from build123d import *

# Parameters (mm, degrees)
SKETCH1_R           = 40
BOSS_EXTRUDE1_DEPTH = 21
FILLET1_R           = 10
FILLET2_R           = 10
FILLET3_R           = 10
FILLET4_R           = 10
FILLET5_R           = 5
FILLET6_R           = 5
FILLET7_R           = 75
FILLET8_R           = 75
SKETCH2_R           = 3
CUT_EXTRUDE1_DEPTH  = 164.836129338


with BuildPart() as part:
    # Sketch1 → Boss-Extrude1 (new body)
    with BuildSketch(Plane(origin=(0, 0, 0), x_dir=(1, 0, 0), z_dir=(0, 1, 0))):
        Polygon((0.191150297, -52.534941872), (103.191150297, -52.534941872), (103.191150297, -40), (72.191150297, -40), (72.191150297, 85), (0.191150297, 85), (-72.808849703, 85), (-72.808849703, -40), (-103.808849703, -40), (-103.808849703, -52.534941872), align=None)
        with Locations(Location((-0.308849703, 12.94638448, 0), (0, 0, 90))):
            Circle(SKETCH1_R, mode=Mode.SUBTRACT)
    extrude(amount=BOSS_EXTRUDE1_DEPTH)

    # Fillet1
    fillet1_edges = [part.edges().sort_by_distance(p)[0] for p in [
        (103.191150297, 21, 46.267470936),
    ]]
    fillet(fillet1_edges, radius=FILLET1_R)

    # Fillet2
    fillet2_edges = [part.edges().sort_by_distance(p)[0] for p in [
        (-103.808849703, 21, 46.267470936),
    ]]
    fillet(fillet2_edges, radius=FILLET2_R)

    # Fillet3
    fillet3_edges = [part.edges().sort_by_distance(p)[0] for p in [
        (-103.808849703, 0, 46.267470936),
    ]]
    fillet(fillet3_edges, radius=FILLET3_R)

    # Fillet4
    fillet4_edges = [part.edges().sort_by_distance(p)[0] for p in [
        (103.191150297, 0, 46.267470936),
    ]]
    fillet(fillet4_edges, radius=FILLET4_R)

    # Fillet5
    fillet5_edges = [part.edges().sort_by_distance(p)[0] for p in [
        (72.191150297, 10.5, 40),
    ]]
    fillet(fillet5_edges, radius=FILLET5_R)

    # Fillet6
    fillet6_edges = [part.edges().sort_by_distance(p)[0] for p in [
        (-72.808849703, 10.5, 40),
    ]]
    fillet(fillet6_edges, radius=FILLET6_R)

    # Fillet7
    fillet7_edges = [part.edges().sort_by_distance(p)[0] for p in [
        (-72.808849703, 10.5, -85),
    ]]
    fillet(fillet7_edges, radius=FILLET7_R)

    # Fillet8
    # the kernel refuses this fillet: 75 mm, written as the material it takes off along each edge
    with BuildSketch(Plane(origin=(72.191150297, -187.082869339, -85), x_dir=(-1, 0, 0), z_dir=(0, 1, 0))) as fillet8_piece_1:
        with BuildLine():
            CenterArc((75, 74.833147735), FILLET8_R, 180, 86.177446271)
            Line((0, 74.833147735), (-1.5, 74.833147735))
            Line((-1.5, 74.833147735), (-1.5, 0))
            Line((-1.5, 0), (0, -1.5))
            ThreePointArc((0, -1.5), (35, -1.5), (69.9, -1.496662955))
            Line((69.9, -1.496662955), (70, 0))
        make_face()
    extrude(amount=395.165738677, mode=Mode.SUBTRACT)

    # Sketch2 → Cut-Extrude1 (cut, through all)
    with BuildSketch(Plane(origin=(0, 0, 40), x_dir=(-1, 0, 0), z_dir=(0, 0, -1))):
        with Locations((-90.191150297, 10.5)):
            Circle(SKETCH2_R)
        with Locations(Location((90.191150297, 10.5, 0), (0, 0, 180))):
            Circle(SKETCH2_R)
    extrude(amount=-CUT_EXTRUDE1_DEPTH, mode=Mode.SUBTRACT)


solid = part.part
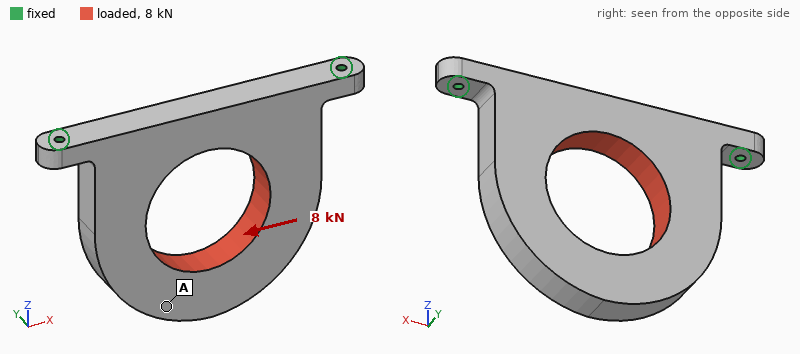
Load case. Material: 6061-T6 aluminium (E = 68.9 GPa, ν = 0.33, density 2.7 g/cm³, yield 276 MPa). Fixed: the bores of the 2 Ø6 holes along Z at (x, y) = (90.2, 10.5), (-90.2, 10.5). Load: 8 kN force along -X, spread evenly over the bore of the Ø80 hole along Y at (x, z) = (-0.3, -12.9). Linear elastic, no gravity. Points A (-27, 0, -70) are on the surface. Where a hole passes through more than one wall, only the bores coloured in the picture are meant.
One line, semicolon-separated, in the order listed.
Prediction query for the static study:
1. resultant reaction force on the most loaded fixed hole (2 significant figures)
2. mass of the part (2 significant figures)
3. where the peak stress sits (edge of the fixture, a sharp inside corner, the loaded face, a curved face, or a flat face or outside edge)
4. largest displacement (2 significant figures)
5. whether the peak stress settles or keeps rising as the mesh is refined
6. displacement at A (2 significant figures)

5.0 kN; 750 g; edge of the fixture; 68 µm; keeps rising; 67 µm
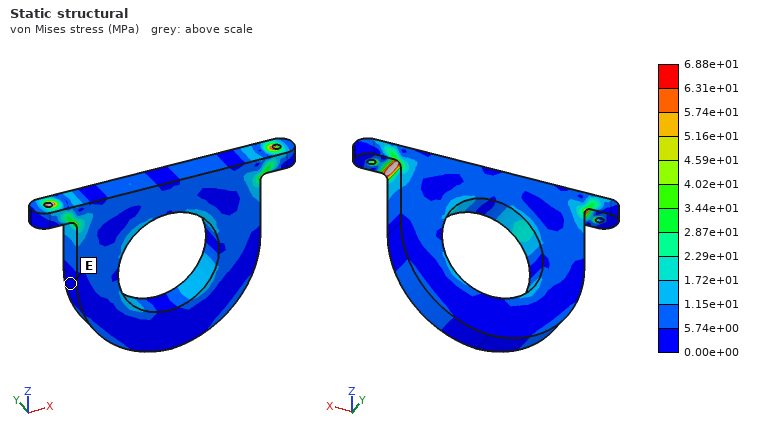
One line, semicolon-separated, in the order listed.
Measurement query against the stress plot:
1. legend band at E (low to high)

0.00e+00 to 5.74e+00 MPa
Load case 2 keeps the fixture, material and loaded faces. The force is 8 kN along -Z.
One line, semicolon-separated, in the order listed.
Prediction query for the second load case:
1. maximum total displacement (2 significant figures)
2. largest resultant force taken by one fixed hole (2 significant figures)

53 µm; 4.7 kN
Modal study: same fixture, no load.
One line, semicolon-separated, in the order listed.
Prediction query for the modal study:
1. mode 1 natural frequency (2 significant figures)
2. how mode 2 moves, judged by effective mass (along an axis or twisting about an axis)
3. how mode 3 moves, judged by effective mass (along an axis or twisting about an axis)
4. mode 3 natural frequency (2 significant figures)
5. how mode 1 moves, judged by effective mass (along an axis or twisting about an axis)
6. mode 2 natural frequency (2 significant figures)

380 Hz; twisting about Z; along Y; 2200 Hz; along Y; 1800 Hz
